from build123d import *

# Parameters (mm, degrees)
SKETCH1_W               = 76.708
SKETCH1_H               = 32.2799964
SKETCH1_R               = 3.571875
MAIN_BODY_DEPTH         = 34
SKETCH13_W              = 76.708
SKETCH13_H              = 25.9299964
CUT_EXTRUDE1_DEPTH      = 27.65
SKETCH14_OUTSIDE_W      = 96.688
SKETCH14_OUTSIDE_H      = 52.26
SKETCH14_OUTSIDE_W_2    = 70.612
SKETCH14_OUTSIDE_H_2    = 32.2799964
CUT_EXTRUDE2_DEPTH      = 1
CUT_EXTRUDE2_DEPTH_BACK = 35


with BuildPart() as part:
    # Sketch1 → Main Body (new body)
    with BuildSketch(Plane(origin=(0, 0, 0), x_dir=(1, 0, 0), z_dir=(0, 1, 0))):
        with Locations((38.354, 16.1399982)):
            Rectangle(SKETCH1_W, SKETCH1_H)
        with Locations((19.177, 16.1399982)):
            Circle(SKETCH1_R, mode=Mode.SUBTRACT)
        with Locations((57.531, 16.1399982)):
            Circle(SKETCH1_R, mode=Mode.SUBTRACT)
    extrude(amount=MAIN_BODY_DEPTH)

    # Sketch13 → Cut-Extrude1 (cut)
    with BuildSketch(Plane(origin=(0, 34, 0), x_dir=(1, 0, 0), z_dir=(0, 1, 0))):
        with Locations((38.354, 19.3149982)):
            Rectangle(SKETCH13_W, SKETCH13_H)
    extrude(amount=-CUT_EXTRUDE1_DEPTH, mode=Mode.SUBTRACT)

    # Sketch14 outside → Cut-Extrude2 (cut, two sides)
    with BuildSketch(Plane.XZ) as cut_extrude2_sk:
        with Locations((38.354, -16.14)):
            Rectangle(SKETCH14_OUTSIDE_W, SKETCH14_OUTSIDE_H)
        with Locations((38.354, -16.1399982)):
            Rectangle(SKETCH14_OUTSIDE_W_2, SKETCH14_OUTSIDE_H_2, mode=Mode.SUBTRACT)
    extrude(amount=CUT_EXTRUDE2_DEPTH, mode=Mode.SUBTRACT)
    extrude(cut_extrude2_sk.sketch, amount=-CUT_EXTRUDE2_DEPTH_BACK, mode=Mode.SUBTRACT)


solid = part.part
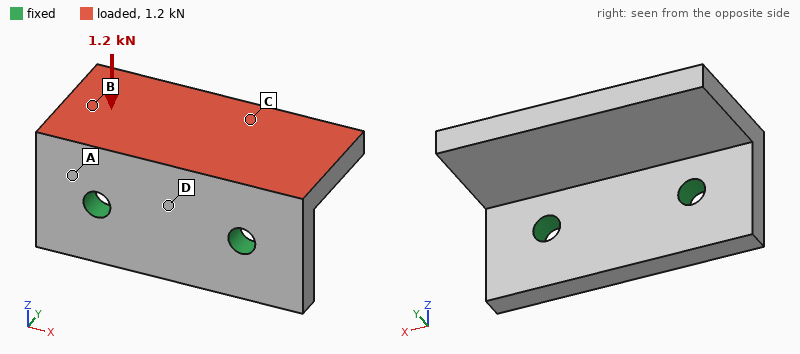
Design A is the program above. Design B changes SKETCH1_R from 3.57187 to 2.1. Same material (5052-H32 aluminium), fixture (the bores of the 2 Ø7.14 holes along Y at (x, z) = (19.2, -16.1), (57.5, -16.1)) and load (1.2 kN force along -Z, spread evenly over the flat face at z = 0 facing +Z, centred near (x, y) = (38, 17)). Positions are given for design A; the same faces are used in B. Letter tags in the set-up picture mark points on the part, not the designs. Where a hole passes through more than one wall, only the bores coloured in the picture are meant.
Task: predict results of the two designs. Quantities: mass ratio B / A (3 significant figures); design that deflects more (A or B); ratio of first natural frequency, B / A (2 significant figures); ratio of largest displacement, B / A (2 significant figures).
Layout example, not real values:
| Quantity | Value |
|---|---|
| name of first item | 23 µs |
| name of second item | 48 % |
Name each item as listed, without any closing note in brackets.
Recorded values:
| Quantity | Value |
|---|---|
| mass ratio B / A | 1.01 |
| design that deflects more | B |
| ratio of first natural frequency, B / A | 0.89 |
| ratio of largest displacement, B / A | 1.2 |
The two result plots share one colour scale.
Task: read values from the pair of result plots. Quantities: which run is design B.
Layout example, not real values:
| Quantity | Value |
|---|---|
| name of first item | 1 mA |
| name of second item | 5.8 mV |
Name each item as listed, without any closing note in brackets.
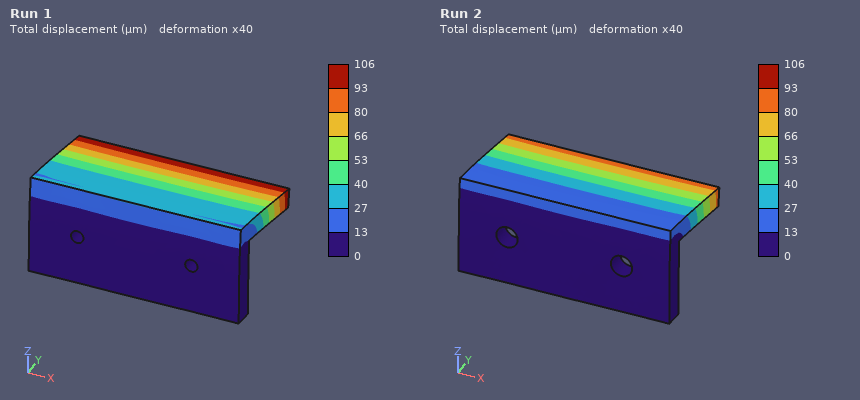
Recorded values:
| Quantity | Value |
|---|---|
| which run is design B | Run 1 |
